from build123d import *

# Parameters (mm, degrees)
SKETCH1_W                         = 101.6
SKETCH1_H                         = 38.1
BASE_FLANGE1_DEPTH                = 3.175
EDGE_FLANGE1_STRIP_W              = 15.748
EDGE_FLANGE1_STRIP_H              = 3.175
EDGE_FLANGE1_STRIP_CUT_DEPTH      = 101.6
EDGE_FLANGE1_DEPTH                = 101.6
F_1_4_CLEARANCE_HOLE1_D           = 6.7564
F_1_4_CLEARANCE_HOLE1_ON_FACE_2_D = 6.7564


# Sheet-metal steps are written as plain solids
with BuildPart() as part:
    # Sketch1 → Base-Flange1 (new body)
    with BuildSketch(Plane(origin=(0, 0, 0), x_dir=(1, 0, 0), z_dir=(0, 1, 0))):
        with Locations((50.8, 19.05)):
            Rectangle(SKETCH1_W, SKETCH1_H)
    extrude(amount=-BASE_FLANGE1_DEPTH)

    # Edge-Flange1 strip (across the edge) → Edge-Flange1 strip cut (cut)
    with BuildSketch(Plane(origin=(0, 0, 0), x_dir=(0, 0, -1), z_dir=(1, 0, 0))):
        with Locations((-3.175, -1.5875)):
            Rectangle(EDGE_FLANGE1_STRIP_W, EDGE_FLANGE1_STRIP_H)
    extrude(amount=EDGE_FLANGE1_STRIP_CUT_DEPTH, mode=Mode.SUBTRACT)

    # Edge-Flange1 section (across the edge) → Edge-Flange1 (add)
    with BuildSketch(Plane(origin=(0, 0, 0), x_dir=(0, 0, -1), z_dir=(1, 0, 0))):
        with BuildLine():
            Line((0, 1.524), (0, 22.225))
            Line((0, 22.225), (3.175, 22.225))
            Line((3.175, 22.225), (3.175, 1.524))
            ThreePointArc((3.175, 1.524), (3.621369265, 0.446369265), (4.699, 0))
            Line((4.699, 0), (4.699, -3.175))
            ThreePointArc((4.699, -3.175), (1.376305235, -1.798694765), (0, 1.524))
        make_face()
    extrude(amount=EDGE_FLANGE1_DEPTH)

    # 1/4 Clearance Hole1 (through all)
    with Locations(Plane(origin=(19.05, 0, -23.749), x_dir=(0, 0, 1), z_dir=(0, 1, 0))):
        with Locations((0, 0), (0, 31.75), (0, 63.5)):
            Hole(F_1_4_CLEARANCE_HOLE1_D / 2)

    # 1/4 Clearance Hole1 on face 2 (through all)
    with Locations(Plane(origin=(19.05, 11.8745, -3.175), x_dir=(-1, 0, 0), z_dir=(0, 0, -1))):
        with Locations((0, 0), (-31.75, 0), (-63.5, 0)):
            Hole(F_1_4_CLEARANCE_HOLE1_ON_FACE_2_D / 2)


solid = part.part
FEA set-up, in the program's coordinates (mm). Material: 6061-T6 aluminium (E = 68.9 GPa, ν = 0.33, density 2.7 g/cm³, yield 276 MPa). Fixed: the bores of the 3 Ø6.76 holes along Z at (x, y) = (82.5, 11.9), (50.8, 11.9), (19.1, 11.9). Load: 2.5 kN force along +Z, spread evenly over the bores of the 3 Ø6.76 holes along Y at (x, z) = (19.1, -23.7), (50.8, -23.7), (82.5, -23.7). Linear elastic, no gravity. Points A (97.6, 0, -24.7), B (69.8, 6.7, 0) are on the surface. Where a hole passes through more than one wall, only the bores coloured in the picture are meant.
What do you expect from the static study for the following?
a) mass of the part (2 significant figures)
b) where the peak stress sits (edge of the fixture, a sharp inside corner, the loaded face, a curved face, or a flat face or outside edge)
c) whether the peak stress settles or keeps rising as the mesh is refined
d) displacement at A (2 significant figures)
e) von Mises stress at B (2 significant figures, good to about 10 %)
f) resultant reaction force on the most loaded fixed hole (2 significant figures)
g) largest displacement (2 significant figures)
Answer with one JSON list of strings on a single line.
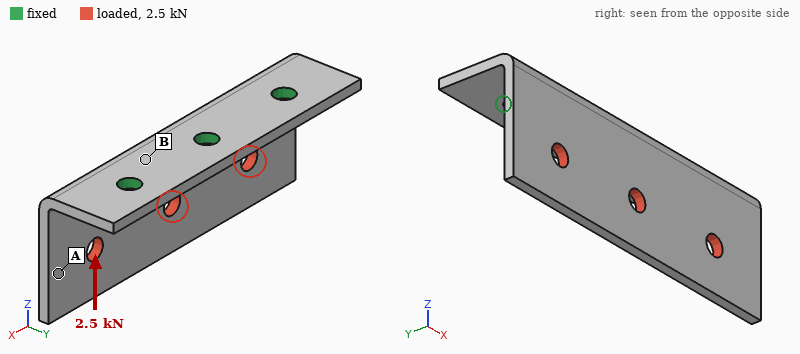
["50 g", "edge of the fixture", "keeps rising", "0.25 mm", "66 MPa", "840 N", "0.40 mm"]
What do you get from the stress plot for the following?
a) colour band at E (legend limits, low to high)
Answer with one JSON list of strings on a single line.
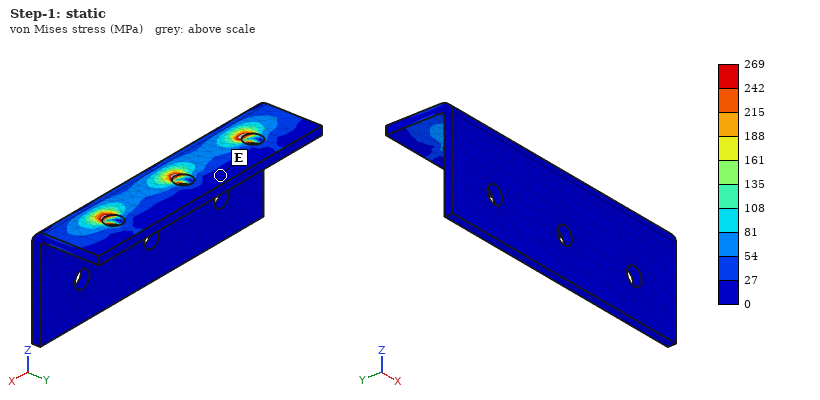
["0 to 27 MPa"]
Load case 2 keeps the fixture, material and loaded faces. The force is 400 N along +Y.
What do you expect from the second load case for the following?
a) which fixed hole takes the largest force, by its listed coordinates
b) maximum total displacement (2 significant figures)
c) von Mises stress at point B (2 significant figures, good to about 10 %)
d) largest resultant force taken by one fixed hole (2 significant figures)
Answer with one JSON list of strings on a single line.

["(50.8, 11.9)", "0.34 mm", "35 MPa", "150 N"]
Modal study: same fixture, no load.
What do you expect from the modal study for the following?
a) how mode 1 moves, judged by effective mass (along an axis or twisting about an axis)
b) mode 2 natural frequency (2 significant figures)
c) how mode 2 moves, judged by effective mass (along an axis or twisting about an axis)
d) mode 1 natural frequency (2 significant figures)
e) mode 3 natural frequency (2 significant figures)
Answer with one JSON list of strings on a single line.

["along Y", "1900 Hz", "twisting about Z", "1300 Hz", "3700 Hz"]
